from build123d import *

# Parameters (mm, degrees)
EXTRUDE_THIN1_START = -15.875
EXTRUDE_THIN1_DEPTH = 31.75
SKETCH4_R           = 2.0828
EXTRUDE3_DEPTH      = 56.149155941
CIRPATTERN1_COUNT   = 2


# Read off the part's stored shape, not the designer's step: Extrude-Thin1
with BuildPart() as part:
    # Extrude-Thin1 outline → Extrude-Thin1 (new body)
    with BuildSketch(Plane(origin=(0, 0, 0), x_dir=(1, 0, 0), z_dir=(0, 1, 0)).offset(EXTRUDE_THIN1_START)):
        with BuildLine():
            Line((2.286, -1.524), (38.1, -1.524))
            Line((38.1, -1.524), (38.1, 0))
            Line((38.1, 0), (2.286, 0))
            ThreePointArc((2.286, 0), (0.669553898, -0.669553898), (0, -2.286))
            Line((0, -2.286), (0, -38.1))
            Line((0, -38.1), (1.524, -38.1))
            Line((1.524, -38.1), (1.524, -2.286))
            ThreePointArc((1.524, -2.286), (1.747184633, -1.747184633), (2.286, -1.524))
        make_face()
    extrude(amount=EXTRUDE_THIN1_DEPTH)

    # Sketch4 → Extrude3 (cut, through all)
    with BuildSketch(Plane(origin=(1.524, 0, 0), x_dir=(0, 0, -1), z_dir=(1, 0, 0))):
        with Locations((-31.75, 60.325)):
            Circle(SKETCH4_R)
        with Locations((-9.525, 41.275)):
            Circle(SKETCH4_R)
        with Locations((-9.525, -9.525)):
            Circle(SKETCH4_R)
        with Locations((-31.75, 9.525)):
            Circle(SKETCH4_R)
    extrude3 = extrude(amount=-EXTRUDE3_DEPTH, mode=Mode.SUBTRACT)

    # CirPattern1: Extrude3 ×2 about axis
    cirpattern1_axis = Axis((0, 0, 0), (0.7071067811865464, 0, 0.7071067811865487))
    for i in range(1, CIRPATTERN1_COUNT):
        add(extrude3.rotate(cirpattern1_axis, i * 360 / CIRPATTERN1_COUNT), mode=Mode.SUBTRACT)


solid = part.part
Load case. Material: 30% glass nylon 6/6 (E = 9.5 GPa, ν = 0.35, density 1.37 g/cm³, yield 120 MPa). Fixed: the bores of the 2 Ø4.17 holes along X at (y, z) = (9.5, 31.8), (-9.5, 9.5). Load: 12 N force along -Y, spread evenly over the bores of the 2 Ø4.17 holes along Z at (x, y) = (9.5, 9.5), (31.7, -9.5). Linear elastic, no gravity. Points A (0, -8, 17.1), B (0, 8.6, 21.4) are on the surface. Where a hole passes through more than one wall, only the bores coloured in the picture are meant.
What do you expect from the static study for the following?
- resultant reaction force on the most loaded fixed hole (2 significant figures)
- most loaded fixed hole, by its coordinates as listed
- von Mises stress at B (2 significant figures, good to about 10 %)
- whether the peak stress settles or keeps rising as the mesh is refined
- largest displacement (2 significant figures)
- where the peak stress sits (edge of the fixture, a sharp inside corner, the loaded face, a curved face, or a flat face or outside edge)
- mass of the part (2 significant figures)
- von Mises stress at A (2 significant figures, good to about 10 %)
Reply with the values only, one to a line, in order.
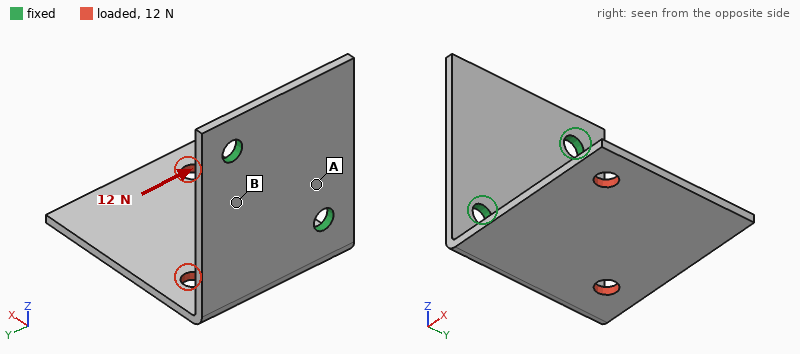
13 N
(-9.5, 9.5)
5.7 MPa
keeps rising
0.67 mm
edge of the fixture
4.8 g
2.5 MPa
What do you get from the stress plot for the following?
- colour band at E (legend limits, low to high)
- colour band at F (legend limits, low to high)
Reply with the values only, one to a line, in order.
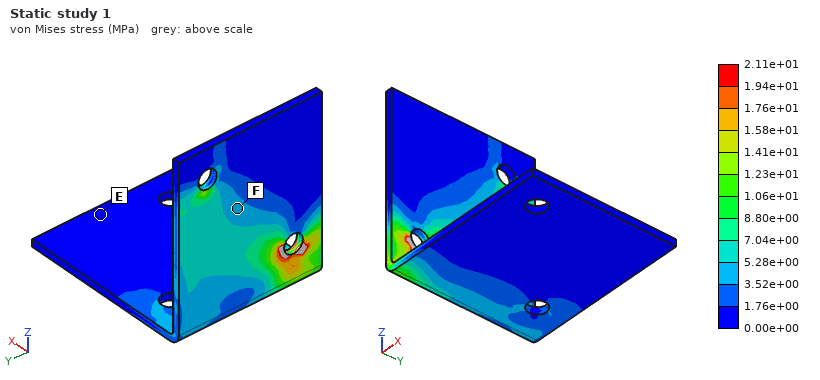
0.00e+00 to 1.76e+00 MPa
3.52e+00 to 5.28e+00 MPa
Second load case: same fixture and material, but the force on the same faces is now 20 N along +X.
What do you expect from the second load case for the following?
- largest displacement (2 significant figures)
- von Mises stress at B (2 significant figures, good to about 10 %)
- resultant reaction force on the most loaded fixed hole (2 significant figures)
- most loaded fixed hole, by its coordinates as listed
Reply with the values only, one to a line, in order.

0.71 mm
5.1 MPa
20 N
(-9.5, 9.5)
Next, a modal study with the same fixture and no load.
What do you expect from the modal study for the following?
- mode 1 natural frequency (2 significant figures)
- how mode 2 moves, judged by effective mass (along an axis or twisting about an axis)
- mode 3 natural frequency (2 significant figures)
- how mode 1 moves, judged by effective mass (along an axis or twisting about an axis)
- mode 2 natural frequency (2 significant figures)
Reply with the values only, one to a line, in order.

330 Hz
along Y
1200 Hz
along Z
560 Hz
